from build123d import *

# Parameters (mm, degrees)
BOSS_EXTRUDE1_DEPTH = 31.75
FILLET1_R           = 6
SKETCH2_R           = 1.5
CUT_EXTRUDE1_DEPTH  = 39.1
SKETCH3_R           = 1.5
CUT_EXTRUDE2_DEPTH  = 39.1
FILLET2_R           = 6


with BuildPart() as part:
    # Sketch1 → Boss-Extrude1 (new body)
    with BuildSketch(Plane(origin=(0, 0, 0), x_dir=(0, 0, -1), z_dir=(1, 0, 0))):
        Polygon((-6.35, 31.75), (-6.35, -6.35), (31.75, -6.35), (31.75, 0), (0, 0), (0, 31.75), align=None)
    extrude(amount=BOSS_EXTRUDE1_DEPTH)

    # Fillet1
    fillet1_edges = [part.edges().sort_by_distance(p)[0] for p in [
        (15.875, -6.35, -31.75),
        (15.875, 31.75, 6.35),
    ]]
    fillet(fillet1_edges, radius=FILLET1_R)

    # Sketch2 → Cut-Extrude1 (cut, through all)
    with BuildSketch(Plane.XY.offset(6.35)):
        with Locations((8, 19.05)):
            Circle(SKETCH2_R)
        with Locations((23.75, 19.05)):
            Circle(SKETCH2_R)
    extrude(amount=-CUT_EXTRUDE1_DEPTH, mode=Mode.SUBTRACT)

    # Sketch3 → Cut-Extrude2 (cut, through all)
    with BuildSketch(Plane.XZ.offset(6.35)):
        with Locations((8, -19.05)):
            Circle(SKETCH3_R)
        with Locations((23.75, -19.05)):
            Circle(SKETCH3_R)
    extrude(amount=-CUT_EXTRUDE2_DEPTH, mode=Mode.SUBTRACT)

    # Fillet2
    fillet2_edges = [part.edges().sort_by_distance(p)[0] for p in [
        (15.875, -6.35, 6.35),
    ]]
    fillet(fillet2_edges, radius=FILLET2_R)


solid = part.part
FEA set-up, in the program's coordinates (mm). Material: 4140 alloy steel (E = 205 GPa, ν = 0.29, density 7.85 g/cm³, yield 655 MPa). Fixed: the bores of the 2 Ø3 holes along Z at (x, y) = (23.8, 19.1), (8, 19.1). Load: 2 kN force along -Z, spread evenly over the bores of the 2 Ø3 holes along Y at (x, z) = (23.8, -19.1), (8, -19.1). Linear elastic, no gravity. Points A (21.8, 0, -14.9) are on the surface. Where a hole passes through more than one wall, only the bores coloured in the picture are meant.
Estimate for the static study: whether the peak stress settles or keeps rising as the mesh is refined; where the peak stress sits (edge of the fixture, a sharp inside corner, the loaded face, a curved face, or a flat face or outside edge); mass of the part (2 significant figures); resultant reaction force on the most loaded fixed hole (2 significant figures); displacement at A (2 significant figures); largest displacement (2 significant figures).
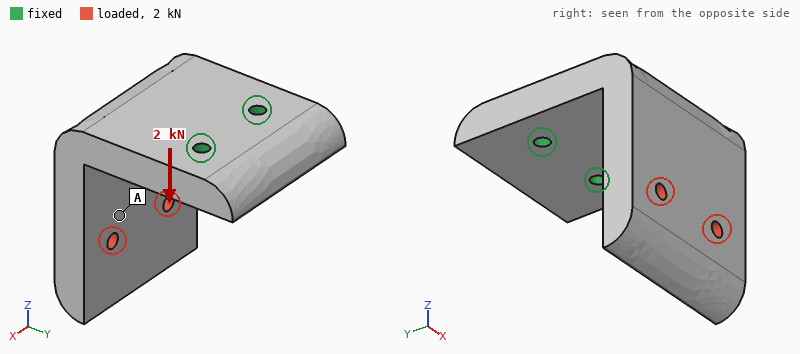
keeps rising
edge of the fixture
100 g
1.0 kN
0.086 mm
0.15 mm
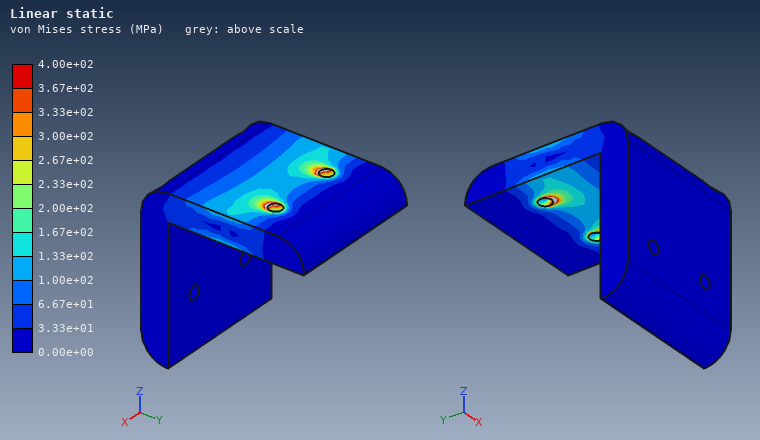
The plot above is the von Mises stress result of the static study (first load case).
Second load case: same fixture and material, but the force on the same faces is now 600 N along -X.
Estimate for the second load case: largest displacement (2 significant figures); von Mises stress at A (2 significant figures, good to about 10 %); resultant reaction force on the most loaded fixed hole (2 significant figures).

40 µm
11 MPa
1.0 kN
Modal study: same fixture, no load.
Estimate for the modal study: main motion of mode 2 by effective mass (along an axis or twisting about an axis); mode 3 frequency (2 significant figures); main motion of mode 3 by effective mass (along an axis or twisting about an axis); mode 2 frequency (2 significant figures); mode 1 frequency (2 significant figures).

along X
6200 Hz
along Z
3600 Hz
2200 Hz
